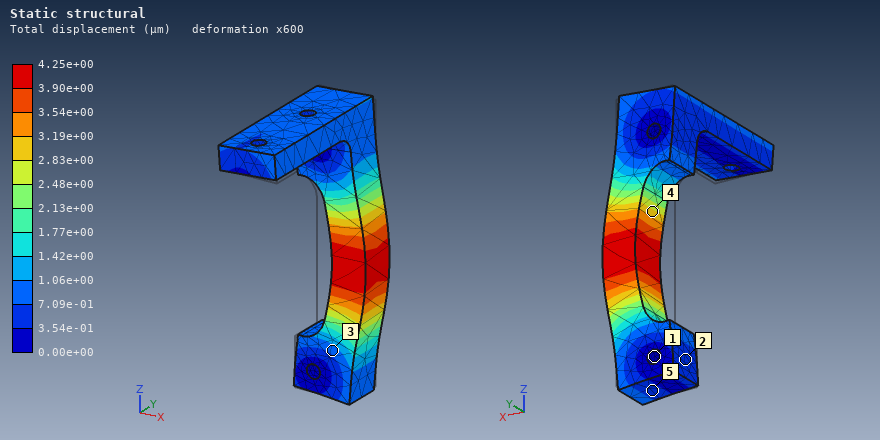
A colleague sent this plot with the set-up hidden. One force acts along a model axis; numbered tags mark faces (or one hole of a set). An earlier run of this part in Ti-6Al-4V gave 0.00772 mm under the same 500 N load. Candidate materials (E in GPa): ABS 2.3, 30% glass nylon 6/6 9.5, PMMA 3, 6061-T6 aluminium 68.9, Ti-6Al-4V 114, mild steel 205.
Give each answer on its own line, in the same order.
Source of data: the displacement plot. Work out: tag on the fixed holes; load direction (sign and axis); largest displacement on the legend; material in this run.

1
+X
4.25e+00 µm
mild steel
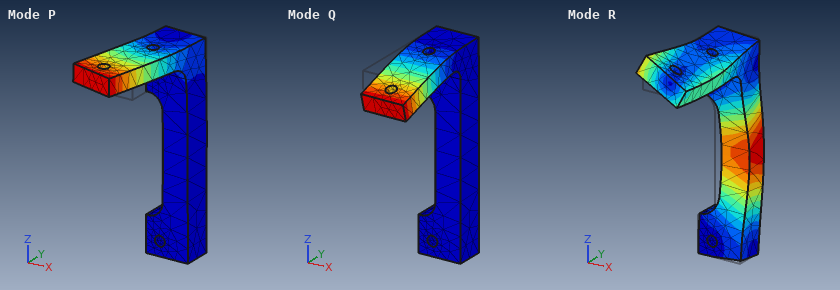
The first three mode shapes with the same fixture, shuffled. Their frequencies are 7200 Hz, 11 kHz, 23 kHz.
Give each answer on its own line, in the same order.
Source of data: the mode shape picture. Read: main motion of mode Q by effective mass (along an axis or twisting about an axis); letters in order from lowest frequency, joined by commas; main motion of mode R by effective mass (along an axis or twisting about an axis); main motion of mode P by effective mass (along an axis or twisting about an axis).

along Z
Q, P, R
along Y
along X
